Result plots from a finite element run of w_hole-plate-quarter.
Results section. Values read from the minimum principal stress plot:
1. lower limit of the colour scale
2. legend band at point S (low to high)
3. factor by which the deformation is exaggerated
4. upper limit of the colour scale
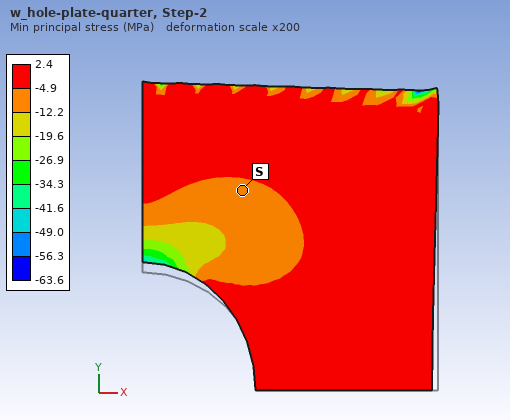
-63.6 MPa
-12.2 to -4.9 MPa
200
2.4 MPa
